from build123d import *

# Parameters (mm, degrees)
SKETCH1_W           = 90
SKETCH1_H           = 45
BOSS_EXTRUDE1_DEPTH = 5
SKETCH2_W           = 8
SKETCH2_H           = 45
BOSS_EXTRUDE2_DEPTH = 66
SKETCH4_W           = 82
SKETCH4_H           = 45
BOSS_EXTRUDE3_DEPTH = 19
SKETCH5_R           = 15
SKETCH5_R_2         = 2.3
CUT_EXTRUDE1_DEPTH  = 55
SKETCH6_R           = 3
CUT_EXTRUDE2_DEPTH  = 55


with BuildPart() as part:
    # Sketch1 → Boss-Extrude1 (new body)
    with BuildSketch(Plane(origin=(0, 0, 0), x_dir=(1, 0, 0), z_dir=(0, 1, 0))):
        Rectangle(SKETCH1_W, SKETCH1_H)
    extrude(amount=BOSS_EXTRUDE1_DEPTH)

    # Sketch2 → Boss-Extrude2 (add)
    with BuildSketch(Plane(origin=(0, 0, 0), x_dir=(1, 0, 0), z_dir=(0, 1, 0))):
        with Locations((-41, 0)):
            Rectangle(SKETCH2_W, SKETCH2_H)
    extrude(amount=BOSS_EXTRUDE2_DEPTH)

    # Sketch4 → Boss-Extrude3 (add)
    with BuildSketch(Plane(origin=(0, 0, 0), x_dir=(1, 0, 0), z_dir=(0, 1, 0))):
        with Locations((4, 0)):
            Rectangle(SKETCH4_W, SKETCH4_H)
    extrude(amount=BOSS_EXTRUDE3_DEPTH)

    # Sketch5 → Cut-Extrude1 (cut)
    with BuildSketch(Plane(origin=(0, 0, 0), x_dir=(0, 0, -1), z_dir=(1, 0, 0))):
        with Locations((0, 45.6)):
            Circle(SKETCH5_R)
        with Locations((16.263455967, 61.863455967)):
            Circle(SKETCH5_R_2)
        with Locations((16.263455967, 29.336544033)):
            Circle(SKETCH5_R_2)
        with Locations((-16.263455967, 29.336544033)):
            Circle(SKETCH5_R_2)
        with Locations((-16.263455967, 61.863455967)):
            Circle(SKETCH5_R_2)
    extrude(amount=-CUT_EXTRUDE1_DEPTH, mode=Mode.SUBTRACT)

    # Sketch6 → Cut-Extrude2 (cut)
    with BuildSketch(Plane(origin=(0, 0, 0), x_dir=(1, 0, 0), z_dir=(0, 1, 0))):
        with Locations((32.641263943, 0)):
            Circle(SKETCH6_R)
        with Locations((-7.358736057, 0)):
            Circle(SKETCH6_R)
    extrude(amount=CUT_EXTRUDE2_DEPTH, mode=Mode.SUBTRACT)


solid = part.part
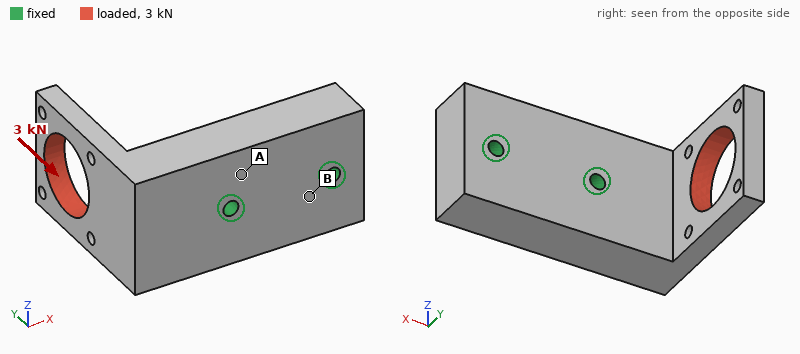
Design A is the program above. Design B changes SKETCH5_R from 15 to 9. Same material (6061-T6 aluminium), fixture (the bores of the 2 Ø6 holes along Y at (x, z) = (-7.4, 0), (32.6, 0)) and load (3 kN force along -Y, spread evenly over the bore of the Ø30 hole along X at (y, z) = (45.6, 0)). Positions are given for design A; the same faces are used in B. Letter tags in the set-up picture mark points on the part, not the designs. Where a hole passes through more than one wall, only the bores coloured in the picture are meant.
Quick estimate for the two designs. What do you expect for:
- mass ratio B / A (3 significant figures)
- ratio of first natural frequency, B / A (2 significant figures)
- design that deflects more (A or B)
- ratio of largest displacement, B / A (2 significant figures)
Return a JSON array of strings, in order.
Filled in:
["1.04", "0.99", "A", "0.90"]
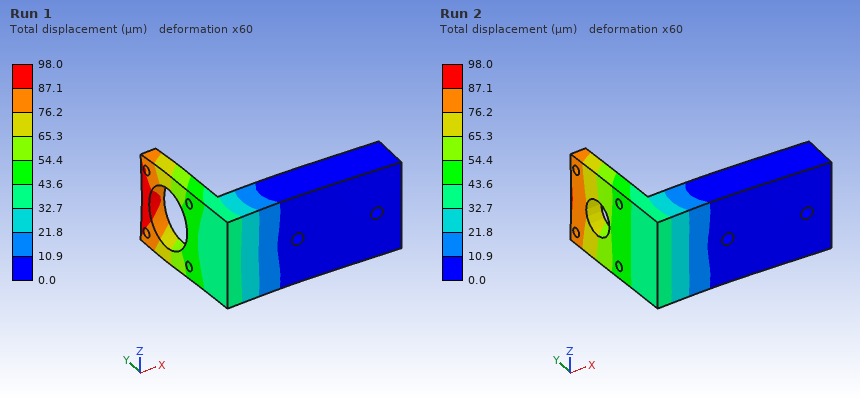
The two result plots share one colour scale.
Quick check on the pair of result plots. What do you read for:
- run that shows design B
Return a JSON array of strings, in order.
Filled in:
["Run 2"]
